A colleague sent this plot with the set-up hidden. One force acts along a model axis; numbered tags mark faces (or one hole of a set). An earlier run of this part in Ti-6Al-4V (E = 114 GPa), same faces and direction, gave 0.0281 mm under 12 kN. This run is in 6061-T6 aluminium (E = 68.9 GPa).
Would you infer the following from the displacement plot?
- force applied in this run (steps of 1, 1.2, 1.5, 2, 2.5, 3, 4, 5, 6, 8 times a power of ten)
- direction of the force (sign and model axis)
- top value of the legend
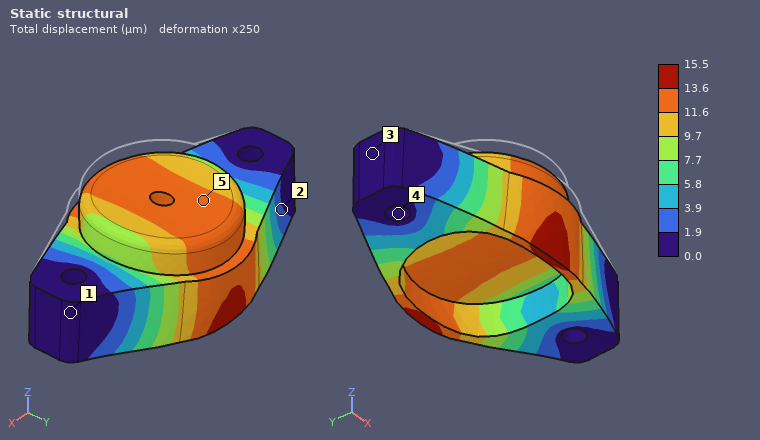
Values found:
4 kN
-Z
15.5 µm
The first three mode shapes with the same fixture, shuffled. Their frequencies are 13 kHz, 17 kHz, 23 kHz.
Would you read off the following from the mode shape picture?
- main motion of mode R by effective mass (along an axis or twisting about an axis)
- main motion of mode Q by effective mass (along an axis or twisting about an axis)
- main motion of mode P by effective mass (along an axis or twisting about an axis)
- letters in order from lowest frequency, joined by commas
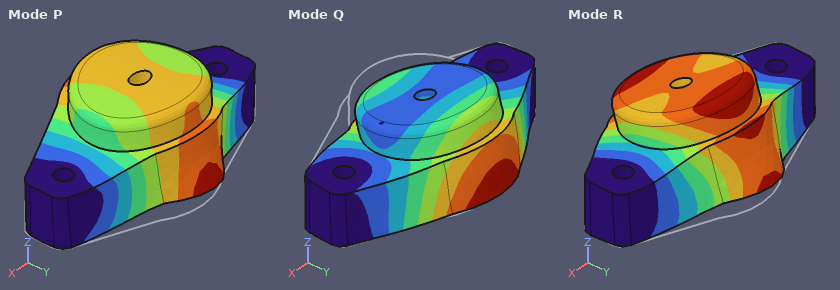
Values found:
along Y
along Y
along Z
R, P, Q
